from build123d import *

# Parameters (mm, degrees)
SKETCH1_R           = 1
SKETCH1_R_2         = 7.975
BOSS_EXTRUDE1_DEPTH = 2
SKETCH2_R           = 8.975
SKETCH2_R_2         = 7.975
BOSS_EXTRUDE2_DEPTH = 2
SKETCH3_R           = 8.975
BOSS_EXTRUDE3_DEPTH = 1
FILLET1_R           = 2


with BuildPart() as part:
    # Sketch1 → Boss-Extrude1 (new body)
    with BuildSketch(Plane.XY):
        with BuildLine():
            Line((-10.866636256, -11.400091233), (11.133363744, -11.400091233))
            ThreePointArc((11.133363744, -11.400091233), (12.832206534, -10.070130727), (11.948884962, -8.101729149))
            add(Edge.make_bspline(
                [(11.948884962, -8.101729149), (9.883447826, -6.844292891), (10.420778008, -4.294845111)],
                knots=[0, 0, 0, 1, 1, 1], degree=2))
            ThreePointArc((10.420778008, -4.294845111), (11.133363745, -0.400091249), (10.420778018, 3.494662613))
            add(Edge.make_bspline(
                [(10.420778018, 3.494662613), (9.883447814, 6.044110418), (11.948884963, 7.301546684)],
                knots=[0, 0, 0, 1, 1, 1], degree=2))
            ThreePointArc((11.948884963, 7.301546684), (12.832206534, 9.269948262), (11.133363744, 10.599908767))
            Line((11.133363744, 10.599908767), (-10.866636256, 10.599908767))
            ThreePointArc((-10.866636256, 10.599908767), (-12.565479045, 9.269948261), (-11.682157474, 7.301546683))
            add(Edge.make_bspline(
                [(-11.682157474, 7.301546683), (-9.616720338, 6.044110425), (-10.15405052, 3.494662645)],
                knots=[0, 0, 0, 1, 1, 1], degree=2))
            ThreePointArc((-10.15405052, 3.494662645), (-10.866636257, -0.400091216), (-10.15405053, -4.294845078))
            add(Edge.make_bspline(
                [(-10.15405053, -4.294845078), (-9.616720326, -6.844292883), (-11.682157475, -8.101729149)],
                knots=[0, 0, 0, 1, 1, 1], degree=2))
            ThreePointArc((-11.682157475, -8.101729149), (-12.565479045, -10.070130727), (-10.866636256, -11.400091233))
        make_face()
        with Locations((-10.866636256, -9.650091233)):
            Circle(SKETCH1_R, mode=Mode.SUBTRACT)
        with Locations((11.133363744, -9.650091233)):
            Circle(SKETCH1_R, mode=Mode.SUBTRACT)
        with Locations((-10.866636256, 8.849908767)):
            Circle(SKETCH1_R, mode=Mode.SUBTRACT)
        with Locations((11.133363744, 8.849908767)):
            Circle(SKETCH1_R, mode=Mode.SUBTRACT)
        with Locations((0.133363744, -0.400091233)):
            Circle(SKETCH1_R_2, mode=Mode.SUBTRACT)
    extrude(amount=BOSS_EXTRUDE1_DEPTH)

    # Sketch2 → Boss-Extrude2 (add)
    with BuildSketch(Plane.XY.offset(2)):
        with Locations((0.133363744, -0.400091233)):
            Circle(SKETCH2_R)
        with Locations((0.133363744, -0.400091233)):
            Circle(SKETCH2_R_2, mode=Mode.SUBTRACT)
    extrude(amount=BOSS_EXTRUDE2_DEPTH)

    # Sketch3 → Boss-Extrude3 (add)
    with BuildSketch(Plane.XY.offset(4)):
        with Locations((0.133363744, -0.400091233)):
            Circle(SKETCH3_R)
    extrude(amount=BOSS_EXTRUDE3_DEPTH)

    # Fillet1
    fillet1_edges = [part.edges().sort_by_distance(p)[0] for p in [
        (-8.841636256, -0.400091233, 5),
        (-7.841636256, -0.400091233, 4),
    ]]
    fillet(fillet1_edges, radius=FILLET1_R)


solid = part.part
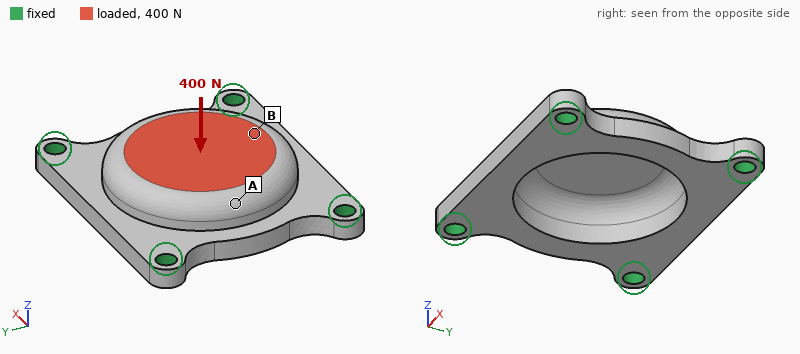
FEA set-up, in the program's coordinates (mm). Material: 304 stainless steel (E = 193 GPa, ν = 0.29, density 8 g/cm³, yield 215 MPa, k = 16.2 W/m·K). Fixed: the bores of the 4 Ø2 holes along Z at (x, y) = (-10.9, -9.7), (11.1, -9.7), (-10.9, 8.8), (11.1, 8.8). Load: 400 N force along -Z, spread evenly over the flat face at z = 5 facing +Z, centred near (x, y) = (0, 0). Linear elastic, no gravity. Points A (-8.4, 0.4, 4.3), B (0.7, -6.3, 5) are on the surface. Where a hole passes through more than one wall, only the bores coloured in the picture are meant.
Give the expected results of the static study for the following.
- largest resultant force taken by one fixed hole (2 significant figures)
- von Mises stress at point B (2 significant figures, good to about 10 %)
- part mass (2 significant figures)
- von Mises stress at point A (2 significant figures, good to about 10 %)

140 N
49 MPa
7.3 g
18 MPa
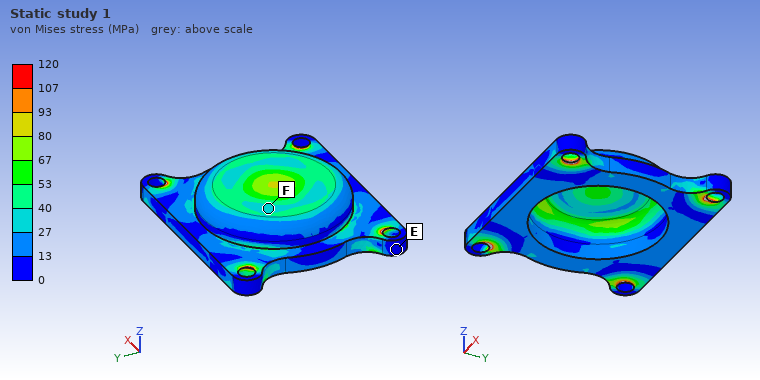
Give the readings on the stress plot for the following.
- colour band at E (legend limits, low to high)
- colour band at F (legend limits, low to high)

0 to 13 MPa
27 to 40 MPa
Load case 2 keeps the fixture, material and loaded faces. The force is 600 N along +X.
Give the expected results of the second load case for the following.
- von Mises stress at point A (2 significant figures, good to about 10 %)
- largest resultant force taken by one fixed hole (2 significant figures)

16 MPa
170 N
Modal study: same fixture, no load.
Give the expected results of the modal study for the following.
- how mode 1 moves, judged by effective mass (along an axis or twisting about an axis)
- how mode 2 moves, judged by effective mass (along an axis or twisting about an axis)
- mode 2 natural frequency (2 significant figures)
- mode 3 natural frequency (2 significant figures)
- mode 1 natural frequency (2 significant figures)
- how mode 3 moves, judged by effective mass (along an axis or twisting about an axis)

along Z
twisting about X
25 kHz
30 kHz
21 kHz
twisting about Y
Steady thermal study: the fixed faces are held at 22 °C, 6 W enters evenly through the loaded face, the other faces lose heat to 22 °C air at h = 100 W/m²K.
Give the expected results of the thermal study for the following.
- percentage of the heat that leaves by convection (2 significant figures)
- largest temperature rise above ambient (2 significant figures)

51 %
64 K
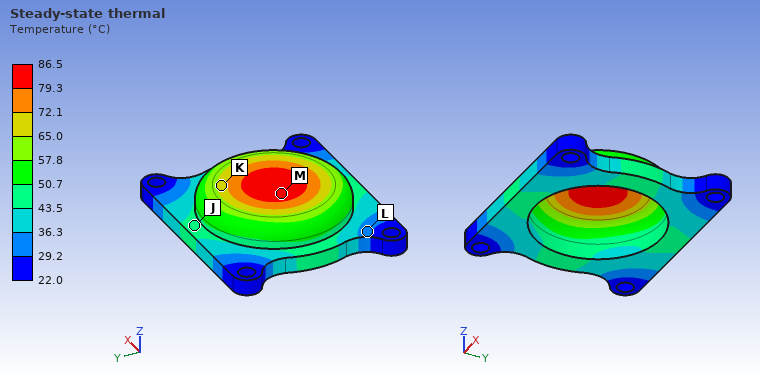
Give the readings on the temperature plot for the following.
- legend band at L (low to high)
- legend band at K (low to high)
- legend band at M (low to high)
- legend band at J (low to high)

29.2 to 36.3 °C
65.0 to 72.1 °C
79.3 to 86.5 °C
43.5 to 50.7 °C
